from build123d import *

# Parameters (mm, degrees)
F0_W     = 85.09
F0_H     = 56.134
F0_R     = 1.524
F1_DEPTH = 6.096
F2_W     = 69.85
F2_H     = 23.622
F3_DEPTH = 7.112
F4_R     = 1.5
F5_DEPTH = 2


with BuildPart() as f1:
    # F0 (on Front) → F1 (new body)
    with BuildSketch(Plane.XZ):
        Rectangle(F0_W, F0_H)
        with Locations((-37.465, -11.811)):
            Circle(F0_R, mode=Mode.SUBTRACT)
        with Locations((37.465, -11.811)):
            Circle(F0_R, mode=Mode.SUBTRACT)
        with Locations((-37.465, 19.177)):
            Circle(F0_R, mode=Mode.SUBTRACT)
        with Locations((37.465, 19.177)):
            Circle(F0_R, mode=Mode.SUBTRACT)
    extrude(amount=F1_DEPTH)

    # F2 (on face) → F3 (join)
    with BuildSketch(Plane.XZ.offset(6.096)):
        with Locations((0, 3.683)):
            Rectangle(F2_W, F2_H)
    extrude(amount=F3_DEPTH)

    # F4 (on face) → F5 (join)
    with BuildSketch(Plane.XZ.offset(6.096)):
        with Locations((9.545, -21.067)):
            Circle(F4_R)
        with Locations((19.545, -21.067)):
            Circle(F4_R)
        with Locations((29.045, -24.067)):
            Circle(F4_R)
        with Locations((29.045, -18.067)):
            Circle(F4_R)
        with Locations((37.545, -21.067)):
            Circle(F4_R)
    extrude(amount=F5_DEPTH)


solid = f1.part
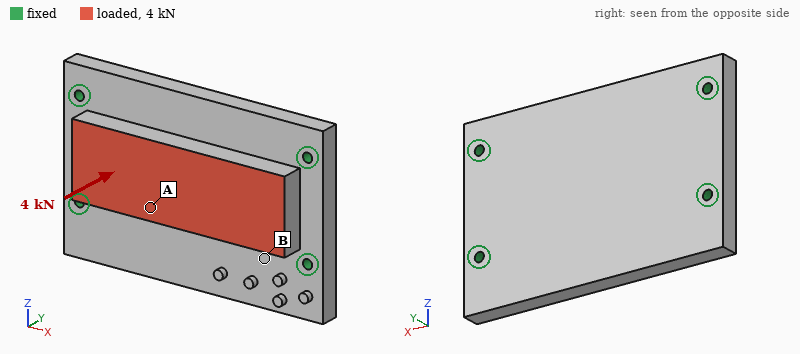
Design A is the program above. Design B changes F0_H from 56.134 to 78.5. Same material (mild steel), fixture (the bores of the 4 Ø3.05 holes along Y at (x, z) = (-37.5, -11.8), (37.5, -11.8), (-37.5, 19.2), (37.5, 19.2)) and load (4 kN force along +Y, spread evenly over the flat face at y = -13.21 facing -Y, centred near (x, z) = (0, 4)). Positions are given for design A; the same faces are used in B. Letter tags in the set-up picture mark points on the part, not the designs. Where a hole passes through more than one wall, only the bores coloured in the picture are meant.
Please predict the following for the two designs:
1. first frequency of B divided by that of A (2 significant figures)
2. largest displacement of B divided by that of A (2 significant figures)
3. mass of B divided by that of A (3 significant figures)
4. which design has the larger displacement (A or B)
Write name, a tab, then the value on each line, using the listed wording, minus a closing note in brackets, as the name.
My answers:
first frequency of B divided by that of A	0.72
largest displacement of B divided by that of A	0.91
mass of B divided by that of A	1.28
which design has the larger displacement	A
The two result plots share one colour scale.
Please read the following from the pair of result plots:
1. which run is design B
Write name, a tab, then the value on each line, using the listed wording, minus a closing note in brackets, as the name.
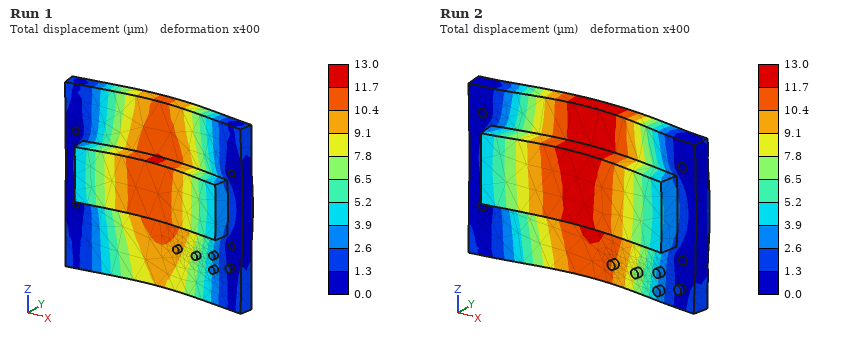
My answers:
which run is design B	Run 1
